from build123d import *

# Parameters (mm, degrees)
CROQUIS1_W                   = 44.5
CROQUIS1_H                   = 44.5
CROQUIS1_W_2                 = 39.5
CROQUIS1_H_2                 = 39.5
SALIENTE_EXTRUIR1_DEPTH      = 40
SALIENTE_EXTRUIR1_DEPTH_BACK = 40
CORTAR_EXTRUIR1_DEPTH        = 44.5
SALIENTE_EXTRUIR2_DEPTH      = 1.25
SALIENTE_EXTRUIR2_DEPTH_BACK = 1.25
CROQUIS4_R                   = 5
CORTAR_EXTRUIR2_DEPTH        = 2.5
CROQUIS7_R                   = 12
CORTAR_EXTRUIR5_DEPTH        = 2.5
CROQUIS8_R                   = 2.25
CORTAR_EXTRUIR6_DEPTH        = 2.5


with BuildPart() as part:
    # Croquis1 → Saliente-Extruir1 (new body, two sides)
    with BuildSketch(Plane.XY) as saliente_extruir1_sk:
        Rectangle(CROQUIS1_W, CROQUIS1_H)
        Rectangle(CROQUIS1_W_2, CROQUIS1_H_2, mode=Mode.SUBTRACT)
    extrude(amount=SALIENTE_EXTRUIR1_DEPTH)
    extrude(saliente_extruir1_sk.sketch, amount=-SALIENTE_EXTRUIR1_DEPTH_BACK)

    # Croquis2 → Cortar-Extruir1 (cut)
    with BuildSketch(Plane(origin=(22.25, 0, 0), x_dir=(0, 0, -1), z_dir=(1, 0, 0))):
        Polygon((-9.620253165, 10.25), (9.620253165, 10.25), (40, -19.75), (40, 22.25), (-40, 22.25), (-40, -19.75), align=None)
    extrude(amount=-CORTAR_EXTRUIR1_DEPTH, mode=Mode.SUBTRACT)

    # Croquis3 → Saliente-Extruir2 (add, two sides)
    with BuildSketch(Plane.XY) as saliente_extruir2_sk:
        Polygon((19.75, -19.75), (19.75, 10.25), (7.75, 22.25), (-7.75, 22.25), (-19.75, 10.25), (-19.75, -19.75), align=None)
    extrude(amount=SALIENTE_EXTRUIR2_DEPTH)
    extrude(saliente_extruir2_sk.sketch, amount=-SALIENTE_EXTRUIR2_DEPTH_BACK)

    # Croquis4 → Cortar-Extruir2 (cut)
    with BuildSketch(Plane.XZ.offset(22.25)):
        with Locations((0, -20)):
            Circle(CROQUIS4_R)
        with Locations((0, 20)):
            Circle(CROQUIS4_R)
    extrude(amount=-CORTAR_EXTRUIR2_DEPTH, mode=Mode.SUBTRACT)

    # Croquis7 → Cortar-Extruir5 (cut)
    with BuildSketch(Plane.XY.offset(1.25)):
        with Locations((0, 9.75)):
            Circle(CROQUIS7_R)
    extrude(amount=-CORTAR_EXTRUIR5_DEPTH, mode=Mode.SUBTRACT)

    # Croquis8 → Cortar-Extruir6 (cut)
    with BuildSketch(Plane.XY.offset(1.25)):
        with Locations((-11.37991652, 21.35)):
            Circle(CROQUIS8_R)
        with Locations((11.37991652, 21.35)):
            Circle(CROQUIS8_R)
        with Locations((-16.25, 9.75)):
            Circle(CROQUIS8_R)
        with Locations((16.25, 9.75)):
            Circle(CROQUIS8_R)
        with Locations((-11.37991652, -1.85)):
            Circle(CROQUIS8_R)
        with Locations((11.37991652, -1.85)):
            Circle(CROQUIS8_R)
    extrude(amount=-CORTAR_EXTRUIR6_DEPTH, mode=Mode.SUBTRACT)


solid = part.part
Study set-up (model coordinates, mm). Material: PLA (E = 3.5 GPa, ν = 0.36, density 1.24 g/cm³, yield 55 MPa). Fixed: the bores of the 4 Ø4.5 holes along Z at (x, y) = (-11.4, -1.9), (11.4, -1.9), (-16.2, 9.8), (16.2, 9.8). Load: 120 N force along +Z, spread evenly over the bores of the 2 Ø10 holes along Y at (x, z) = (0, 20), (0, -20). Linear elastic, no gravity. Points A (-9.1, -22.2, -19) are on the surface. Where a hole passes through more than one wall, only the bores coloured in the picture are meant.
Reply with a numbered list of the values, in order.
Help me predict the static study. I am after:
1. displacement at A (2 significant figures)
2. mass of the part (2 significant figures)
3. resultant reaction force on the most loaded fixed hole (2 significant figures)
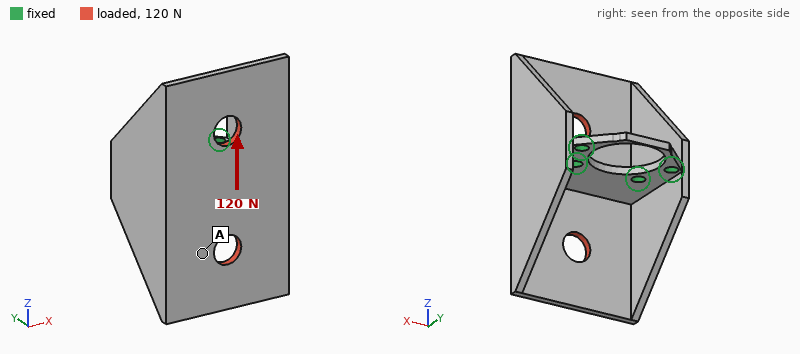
1. 0.37 mm
2. 23 g
3. 110 N
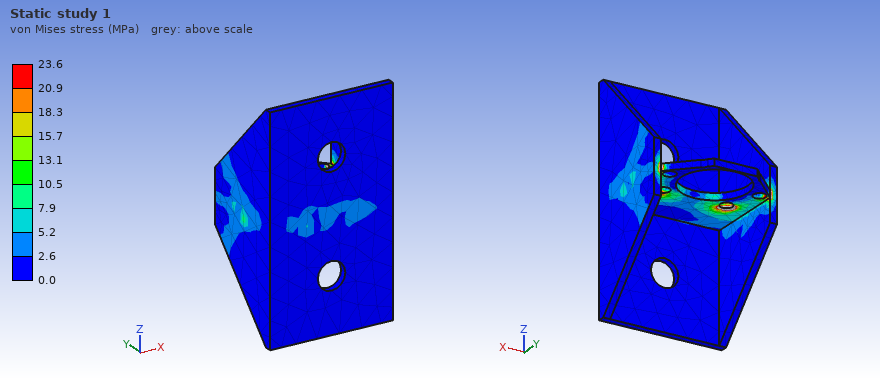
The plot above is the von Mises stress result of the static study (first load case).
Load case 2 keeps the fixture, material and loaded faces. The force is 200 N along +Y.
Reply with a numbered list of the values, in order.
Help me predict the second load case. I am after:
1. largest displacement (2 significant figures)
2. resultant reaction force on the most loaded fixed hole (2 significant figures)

1. 0.45 mm
2. 85 N
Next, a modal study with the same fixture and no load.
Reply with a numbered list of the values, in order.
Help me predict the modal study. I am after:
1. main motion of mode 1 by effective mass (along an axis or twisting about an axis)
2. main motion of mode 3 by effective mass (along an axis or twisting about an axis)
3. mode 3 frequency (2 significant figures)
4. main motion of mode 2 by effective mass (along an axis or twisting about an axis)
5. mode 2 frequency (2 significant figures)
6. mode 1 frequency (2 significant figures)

1. twisting about Y
2. along Z
3. 1500 Hz
4. along Z
5. 620 Hz
6. 500 Hz
